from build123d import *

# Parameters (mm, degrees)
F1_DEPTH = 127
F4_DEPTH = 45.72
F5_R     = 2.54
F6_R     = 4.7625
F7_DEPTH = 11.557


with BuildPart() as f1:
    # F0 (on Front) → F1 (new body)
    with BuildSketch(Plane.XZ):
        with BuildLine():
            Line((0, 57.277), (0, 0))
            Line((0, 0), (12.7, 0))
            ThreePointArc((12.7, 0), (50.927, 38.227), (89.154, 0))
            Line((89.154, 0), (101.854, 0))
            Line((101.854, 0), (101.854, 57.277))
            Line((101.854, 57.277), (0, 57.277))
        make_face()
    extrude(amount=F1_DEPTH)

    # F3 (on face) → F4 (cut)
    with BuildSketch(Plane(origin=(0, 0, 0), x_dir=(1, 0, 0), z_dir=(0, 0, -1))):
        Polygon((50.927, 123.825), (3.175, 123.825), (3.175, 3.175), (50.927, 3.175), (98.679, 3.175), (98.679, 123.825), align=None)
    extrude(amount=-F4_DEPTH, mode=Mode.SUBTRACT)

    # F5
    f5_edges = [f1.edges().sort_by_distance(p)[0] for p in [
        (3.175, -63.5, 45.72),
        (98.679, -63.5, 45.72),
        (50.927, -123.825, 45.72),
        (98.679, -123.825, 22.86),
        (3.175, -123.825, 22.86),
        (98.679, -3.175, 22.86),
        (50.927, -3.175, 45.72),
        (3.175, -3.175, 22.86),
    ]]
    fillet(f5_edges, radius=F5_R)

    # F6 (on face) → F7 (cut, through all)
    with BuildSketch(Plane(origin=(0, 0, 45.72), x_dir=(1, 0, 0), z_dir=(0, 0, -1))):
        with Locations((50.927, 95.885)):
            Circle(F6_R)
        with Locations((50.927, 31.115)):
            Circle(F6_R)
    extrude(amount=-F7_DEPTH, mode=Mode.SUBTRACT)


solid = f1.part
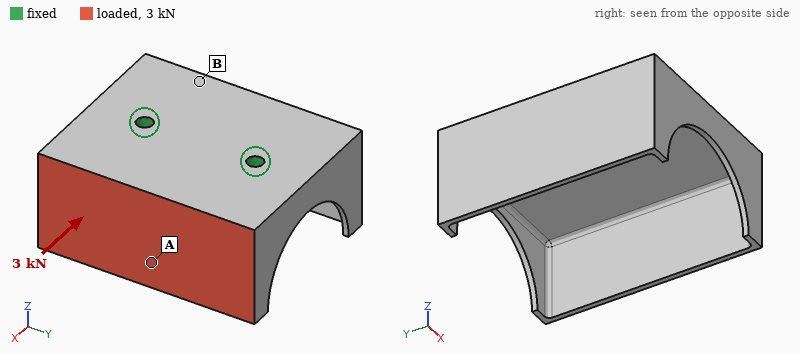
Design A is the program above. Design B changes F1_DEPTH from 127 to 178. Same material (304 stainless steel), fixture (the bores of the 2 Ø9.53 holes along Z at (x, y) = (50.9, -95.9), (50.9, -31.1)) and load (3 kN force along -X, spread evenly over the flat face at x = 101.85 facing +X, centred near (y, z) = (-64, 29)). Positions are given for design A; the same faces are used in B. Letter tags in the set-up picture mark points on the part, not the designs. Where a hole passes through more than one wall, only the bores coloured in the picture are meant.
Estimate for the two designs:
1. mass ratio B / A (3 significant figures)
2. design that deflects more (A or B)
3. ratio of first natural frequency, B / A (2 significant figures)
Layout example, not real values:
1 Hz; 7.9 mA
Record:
1.91; A; 0.70
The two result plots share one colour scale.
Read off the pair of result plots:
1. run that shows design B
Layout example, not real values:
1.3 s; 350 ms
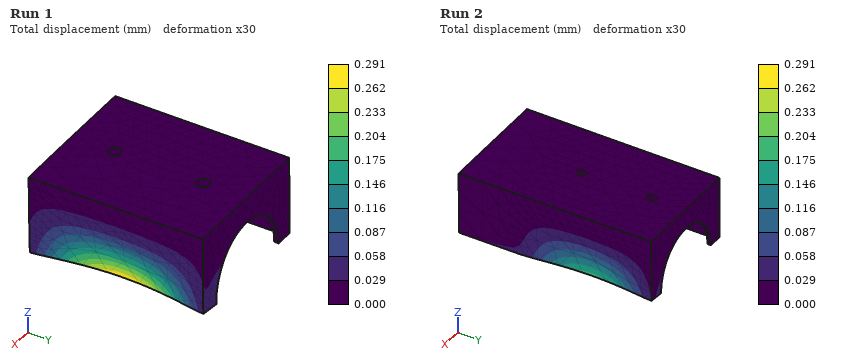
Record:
Run 2
